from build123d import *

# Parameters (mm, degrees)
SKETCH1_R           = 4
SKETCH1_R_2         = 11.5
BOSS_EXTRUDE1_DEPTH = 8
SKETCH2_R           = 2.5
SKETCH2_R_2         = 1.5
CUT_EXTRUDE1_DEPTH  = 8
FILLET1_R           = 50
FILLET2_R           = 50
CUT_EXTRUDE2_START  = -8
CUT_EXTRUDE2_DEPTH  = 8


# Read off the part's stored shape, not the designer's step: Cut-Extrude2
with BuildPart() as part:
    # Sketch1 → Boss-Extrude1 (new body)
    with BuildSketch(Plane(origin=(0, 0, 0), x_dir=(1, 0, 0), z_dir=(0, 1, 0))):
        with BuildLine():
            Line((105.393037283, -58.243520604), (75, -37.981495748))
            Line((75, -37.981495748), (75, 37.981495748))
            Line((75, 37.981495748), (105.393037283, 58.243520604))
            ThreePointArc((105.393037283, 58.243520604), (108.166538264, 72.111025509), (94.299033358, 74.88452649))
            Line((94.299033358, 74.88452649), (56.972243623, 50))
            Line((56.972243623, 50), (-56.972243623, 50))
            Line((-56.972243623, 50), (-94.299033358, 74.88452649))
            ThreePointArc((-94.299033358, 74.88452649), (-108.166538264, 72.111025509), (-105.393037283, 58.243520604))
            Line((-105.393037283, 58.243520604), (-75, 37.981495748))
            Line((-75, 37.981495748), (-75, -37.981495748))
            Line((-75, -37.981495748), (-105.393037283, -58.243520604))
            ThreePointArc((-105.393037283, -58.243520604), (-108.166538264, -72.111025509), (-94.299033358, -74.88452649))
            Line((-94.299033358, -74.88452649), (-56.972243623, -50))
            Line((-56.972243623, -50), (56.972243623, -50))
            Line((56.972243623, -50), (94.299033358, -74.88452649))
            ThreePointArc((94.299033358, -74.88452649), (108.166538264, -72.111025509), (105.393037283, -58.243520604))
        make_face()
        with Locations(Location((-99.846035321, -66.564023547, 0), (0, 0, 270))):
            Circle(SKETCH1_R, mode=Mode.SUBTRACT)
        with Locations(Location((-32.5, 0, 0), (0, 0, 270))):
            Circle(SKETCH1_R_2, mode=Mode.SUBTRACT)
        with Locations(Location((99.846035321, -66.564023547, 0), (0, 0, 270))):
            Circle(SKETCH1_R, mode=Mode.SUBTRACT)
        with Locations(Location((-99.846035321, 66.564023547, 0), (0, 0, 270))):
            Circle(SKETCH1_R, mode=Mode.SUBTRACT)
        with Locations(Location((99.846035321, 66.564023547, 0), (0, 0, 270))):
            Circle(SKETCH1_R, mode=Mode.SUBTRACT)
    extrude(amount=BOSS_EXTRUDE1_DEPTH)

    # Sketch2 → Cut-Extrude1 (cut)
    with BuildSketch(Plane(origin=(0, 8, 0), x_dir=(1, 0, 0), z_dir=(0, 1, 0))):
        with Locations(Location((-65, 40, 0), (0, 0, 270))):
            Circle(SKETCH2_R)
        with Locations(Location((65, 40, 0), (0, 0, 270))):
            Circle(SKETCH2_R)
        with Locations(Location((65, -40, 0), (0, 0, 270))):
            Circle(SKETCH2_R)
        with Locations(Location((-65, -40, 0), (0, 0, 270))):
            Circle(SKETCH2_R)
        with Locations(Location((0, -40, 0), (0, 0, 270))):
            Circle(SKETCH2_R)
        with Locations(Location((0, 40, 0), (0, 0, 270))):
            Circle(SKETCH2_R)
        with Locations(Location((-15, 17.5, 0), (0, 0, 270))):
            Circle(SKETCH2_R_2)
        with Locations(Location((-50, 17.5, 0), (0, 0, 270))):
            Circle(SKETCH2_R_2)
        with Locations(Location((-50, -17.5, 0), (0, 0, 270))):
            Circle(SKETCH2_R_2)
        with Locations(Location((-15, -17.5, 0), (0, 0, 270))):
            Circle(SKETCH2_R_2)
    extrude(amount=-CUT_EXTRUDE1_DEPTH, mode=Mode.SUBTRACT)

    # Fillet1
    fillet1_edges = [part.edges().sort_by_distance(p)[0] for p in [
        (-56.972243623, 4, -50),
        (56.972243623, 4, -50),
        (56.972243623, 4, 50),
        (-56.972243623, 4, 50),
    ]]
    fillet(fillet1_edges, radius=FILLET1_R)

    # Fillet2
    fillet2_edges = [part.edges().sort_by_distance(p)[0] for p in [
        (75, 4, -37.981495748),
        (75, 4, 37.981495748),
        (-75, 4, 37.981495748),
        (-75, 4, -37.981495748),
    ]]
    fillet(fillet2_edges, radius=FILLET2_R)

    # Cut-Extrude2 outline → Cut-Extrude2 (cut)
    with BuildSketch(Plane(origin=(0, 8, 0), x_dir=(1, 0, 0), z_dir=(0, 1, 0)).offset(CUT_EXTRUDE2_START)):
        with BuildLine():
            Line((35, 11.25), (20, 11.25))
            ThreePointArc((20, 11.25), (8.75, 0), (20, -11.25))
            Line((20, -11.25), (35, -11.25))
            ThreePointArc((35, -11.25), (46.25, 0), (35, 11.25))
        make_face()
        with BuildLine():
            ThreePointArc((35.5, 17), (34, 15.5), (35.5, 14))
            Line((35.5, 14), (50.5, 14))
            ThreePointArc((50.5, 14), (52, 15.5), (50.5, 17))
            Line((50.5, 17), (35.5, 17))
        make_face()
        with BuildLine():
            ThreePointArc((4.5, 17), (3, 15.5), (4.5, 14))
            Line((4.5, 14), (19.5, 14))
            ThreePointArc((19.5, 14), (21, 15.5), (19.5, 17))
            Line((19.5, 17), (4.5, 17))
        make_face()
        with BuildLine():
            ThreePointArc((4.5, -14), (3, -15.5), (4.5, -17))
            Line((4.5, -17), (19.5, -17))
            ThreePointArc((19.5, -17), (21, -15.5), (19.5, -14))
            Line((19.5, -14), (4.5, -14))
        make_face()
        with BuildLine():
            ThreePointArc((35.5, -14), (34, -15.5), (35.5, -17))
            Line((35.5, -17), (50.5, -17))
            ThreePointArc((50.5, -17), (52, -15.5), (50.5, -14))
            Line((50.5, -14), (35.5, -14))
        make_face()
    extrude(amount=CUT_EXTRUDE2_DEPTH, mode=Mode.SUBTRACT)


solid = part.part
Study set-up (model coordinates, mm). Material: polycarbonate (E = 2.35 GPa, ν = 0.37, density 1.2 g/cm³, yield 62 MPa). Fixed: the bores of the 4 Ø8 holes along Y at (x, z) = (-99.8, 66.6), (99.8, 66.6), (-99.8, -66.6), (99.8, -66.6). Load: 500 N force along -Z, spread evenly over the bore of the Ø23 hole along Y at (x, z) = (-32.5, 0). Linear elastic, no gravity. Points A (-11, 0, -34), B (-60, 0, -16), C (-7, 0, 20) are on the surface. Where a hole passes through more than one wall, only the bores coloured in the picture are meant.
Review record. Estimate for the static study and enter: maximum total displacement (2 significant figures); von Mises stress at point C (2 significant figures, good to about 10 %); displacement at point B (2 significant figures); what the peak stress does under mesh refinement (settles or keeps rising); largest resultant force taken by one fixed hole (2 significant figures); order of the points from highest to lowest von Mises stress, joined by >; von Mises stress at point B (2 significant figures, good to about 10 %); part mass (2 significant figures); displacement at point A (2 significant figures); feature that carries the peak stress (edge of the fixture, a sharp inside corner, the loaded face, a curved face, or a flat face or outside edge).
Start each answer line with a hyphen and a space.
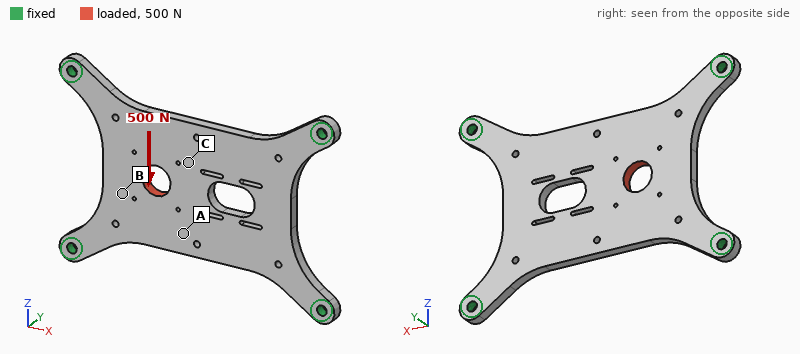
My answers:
- 72 µm
- 0.48 MPa
- 58 µm
- keeps rising
- 240 N
- B > C > A
- 1.0 MPa
- 170 g
- 63 µm
- edge of the fixture
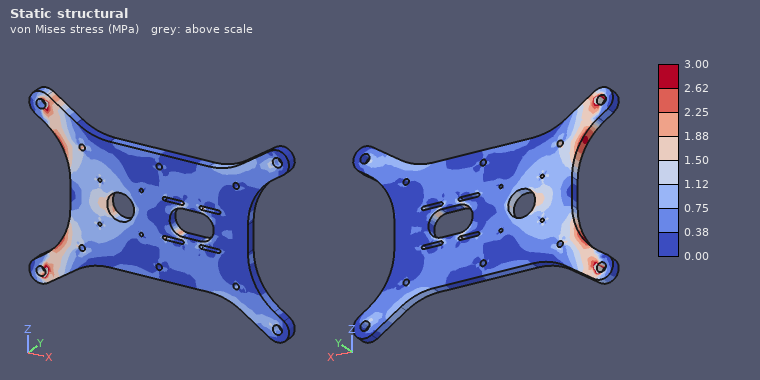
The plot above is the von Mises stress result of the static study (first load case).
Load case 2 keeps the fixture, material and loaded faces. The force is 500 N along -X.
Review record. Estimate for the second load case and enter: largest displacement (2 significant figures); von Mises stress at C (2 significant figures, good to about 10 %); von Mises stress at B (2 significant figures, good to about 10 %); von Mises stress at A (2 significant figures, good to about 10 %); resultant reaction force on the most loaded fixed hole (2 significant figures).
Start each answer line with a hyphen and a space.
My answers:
- 46 µm
- 0.65 MPa
- 0.67 MPa
- 0.30 MPa
- 170 N
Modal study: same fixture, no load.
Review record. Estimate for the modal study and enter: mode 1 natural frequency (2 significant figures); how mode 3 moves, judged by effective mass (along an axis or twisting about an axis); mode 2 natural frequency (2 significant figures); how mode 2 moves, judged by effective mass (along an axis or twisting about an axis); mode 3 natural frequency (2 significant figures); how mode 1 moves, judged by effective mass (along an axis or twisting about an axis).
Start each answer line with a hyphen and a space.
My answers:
- 210 Hz
- twisting about Z
- 440 Hz
- twisting about X
- 510 Hz
- along Y
